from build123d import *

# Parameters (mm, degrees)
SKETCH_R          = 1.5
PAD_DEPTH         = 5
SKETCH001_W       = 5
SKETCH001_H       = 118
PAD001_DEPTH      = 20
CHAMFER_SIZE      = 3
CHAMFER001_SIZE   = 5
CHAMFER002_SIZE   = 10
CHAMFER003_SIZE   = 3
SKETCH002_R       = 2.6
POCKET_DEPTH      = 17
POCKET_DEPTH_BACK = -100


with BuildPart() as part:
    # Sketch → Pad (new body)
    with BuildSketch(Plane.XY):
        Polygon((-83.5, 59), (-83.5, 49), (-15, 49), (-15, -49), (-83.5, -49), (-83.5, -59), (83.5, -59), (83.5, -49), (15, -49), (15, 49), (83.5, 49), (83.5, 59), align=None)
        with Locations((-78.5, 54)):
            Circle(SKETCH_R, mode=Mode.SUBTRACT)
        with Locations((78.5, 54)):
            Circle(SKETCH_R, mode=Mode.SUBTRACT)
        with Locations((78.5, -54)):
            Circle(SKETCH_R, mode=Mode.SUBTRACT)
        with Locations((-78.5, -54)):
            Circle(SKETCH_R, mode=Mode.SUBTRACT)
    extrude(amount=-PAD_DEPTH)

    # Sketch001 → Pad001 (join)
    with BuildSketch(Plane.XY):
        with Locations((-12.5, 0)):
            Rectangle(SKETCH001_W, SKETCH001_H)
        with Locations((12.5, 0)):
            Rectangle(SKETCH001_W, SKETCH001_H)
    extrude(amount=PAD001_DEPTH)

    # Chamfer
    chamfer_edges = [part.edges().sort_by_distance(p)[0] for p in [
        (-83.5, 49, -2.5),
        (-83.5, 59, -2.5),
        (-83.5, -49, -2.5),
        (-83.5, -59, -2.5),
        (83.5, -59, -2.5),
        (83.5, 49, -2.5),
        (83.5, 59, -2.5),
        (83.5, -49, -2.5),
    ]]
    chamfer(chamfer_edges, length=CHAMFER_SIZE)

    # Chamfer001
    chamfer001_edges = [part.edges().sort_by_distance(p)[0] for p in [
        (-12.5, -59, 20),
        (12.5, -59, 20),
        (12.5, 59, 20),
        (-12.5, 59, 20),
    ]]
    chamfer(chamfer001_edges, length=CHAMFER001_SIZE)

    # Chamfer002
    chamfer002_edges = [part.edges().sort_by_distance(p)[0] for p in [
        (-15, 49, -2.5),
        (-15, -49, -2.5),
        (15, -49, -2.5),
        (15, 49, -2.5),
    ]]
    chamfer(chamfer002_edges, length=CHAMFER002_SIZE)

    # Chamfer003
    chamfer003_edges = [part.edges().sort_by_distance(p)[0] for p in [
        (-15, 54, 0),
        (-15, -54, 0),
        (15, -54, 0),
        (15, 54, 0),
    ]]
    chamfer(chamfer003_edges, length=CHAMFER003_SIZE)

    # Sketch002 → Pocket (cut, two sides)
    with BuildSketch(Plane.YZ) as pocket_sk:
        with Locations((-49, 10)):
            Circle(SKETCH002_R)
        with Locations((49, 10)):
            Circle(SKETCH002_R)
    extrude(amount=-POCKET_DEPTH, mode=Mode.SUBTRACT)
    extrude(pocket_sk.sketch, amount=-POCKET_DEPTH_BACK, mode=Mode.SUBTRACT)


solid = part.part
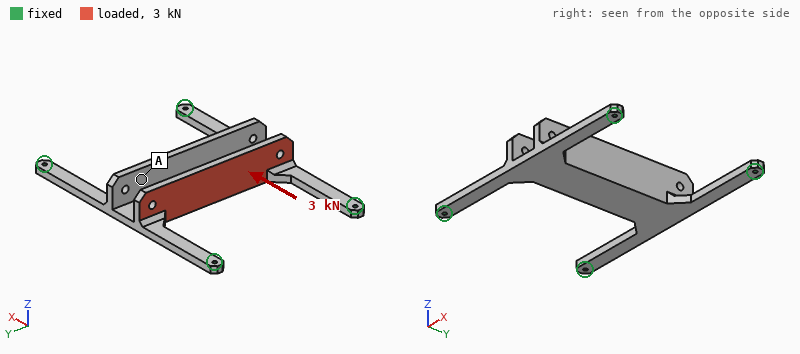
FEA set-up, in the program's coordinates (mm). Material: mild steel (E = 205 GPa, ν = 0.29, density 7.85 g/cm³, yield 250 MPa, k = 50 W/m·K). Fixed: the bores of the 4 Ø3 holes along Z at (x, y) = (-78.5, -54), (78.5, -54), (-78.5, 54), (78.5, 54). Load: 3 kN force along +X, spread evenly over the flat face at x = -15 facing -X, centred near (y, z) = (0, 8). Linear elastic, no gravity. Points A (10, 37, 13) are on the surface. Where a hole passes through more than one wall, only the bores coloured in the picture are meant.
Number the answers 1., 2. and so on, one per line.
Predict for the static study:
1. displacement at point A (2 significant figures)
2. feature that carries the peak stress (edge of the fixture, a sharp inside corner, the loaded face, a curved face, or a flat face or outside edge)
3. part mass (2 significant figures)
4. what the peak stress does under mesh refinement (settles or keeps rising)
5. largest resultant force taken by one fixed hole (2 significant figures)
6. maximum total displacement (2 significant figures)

1. 0.077 mm
2. edge of the fixture
3. 430 g
4. keeps rising
5. 780 N
6. 0.14 mm
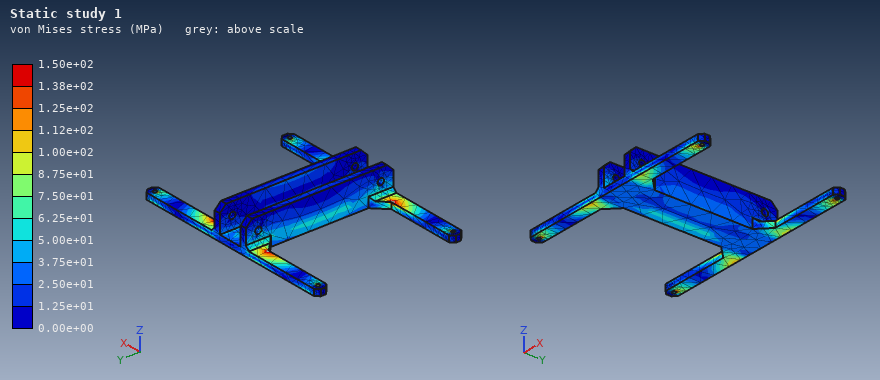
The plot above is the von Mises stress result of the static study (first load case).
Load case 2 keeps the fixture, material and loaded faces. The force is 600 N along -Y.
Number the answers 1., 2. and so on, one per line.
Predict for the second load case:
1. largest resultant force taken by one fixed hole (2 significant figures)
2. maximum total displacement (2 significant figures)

1. 220 N
2. 64 µm
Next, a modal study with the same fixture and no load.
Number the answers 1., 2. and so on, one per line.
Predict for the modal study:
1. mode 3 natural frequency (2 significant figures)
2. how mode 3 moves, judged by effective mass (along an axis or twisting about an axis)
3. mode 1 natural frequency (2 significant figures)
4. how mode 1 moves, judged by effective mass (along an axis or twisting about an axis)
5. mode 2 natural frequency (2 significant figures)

1. 1000 Hz
2. along Y
3. 500 Hz
4. along Z
5. 750 Hz
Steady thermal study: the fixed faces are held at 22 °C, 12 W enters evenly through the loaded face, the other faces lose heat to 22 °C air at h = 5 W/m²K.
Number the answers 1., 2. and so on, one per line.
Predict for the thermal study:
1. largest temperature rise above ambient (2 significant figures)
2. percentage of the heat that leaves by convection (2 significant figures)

1. 58 K
2. 40 %
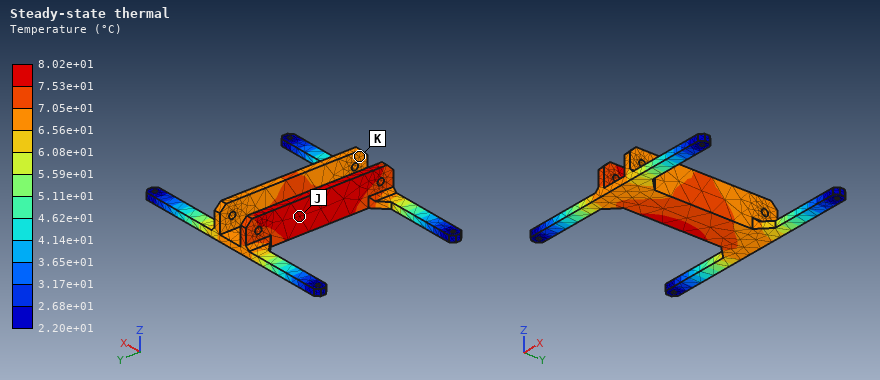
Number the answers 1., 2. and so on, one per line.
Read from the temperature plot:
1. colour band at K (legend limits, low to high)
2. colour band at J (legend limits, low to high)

1. 6.56e+01 to 7.05e+01 °C
2. 7.53e+01 to 8.02e+01 °C
